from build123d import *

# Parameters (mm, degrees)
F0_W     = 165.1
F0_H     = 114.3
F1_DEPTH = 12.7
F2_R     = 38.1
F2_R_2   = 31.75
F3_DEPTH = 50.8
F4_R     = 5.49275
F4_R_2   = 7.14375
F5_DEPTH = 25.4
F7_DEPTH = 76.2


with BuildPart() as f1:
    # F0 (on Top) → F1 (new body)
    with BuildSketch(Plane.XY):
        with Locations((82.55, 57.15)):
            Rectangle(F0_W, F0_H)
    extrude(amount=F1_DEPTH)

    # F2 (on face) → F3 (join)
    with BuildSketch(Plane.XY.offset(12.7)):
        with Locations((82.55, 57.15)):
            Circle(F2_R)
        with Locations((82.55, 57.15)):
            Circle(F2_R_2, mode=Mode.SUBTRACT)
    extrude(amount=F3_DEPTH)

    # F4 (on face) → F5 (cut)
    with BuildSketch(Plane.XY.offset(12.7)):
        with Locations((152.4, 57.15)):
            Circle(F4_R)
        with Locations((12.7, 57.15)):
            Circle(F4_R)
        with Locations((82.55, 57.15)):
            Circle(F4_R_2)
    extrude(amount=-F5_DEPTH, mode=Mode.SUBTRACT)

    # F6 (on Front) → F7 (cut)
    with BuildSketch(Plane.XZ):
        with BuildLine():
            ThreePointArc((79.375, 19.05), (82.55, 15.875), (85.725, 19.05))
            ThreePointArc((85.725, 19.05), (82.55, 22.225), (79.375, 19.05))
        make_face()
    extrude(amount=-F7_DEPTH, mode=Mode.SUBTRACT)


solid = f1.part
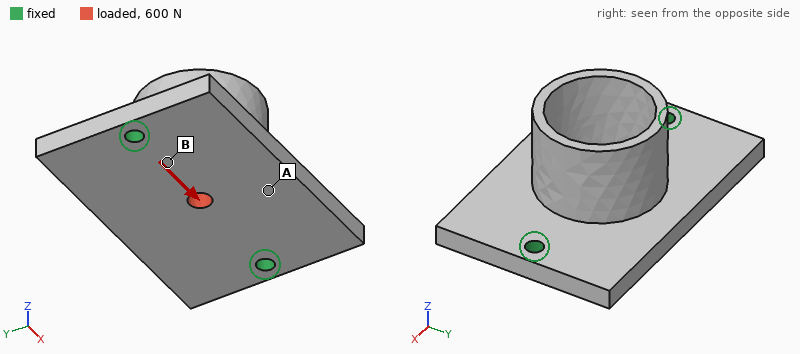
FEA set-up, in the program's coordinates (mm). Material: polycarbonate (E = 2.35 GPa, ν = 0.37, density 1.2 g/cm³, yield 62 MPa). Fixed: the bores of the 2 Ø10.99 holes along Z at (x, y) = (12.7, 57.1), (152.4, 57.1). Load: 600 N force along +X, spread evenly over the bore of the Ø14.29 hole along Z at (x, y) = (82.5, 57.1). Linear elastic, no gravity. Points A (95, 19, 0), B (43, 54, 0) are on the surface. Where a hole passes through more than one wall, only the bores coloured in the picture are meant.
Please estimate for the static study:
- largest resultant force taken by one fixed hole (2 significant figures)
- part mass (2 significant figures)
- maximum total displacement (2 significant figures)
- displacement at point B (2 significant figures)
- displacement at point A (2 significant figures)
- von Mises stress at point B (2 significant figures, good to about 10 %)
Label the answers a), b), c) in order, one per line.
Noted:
a) 300 N
b) 370 g
c) 19 µm
d) 8.4 µm
e) 9.7 µm
f) 0.62 MPa
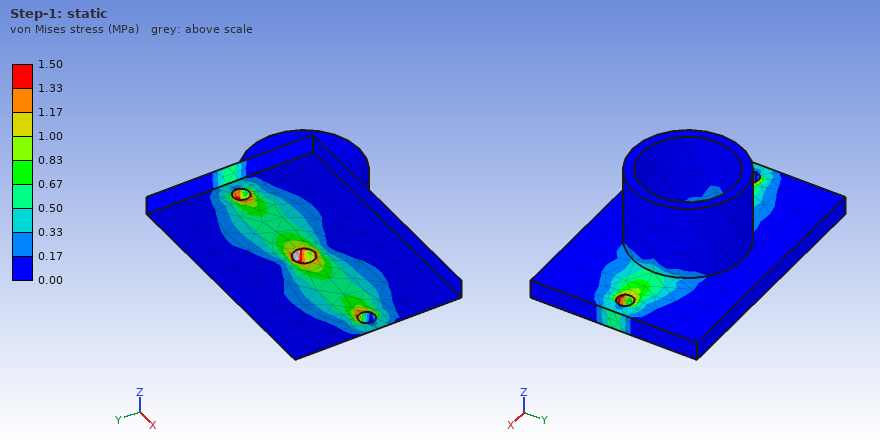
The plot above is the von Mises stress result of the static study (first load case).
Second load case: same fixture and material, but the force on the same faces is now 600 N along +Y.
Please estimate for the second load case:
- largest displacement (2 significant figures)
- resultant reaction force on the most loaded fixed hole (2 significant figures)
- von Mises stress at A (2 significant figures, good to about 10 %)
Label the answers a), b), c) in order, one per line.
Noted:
a) 33 µm
b) 300 N
c) 0.47 MPa
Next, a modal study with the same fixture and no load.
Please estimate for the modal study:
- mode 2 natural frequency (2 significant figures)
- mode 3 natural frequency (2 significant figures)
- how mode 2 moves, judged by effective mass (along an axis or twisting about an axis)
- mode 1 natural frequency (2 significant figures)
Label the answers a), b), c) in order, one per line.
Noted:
a) 630 Hz
b) 1000 Hz
c) along Z
d) 400 Hz
